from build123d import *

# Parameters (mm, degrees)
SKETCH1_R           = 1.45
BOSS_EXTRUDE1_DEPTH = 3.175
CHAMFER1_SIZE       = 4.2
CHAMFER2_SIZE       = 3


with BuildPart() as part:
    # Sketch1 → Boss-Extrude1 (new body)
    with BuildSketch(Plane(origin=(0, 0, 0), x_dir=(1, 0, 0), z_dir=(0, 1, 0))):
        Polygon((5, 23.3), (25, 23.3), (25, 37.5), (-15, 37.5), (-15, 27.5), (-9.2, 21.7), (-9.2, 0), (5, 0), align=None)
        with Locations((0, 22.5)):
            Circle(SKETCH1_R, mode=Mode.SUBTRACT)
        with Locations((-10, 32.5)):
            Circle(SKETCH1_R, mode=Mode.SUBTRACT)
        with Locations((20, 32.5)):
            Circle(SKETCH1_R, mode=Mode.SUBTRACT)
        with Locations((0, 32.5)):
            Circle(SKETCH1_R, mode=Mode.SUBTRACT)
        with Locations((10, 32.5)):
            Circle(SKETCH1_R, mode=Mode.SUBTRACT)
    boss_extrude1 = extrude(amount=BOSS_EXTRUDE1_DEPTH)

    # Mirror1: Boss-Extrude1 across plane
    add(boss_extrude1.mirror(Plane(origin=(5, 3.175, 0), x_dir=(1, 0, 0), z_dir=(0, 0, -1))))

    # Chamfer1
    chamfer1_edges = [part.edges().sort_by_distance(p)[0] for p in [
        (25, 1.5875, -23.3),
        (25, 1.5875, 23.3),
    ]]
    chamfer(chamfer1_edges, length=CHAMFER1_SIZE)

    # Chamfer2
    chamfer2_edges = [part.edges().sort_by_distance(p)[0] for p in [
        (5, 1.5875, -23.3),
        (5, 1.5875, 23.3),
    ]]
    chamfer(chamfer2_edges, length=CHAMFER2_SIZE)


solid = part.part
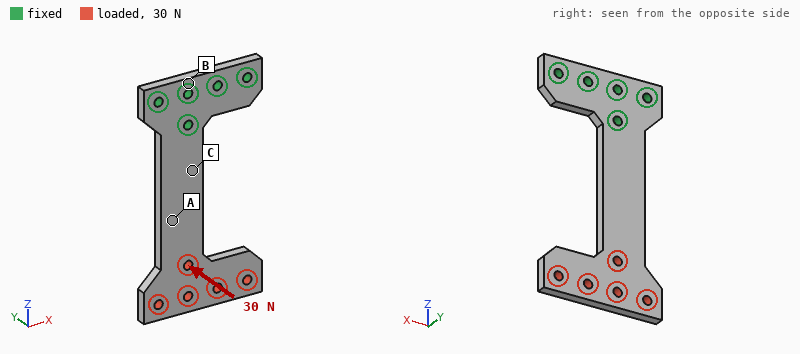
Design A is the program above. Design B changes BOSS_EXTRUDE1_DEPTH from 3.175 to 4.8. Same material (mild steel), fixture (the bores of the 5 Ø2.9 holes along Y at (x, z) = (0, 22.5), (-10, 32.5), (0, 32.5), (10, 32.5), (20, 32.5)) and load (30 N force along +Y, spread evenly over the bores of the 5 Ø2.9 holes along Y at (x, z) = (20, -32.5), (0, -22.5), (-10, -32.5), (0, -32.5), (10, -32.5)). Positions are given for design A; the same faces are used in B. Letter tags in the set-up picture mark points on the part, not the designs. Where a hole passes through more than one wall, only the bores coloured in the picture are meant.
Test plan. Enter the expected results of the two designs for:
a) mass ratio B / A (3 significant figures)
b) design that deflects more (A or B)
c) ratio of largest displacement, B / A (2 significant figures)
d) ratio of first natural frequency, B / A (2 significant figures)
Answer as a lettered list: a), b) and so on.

a) 1.51
b) A
c) 0.30
d) 1.5
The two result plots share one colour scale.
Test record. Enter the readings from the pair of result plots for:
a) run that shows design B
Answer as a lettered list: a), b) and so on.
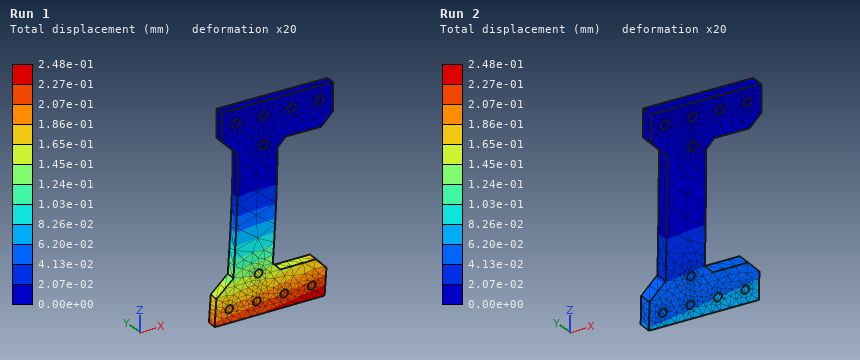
a) Run 2
